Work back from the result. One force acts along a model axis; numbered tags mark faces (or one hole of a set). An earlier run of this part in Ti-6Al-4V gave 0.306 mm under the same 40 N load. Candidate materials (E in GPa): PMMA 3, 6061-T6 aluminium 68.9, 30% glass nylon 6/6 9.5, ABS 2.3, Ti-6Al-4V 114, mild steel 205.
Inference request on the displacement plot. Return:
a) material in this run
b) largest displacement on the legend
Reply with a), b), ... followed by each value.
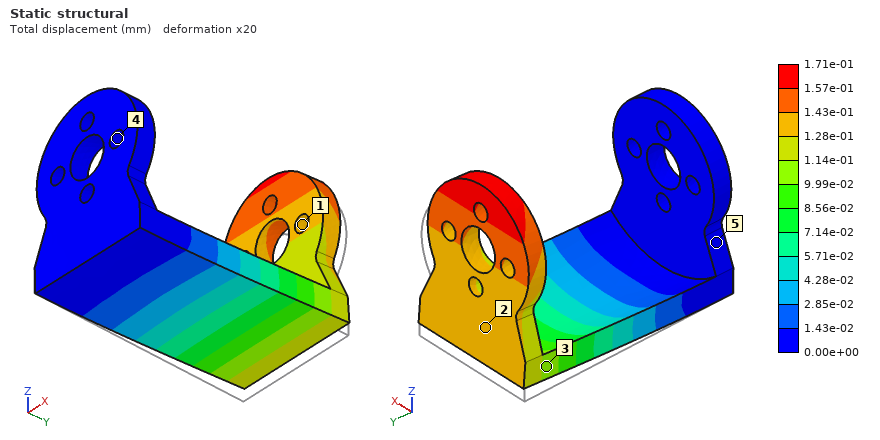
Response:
a) mild steel
b) 1.71e-01 mm
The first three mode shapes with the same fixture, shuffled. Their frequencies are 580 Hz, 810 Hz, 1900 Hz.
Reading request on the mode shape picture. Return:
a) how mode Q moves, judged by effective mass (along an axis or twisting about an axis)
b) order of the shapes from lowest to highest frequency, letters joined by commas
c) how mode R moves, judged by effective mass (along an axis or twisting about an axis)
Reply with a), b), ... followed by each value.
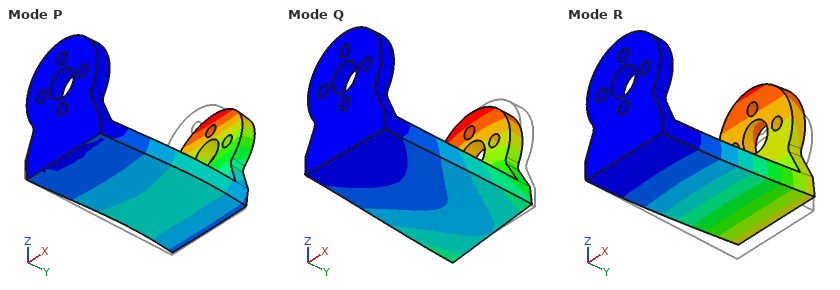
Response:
a) along X
b) R, Q, P
c) along Z
